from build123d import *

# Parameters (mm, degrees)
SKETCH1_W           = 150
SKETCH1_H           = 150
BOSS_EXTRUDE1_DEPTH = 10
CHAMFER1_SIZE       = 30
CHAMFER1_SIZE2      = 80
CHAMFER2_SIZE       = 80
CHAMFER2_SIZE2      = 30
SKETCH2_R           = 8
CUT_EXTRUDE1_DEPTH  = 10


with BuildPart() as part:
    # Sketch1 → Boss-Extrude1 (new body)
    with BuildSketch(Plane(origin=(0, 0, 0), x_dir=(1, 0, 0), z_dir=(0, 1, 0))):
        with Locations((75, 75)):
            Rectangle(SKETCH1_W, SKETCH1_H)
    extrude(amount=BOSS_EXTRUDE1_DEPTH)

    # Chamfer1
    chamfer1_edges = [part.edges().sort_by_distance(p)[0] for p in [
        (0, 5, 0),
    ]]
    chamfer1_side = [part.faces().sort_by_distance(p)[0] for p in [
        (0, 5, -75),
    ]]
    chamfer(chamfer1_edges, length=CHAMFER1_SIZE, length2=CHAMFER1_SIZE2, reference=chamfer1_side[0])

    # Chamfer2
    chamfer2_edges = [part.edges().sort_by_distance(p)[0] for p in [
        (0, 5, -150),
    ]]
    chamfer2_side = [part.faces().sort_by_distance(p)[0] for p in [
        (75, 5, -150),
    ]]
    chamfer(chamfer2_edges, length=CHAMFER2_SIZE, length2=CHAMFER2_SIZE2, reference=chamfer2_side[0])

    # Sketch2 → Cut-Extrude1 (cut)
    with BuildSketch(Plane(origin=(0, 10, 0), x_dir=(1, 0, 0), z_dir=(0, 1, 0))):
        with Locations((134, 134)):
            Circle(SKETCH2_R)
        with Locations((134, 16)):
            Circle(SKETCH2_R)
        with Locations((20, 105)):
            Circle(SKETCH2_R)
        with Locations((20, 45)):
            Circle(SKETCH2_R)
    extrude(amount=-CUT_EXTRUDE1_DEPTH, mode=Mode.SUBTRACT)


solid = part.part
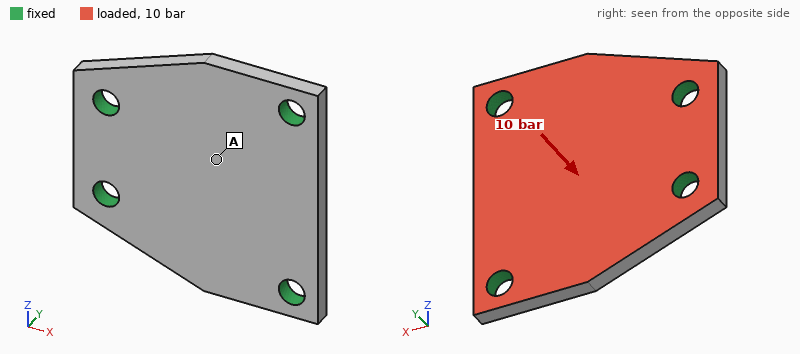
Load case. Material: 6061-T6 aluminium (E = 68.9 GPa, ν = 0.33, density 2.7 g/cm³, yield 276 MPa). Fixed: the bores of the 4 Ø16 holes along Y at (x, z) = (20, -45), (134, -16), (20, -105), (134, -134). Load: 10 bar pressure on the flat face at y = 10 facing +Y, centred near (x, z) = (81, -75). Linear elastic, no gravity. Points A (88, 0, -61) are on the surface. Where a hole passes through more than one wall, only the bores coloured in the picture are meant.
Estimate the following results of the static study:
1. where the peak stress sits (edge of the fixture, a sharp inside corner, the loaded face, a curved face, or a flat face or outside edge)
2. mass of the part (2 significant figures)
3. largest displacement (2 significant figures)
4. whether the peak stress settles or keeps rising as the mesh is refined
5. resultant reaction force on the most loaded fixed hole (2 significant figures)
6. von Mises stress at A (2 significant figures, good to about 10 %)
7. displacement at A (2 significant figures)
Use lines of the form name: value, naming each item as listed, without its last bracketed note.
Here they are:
where the peak stress sits: edge of the fixture
mass of the part: 520 g
largest displacement: 0.11 mm
whether the peak stress settles or keeps rising as the mesh is refined: keeps rising
resultant reaction force on the most loaded fixed hole: 5.1 kN
von Mises stress at A: 28 MPa
displacement at A: 0.11 mm
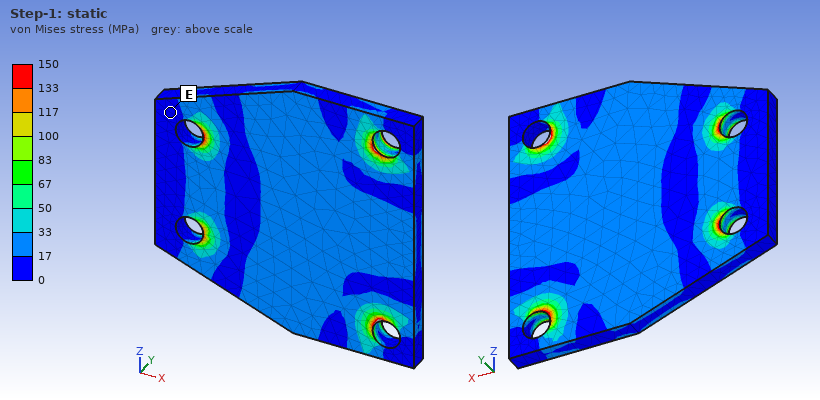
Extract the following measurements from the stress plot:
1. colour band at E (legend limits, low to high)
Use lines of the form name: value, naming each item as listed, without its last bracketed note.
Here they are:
colour band at E: 0 to 17 MPa
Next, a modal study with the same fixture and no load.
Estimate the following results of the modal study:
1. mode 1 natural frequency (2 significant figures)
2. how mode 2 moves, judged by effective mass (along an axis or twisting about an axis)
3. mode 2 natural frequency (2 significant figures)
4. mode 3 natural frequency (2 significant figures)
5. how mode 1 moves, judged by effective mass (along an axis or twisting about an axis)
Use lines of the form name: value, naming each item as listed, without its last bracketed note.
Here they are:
mode 1 natural frequency: 3500 Hz
how mode 2 moves, judged by effective mass: twisting about X
mode 2 natural frequency: 4200 Hz
mode 3 natural frequency: 4500 Hz
how mode 1 moves, judged by effective mass: along Y
